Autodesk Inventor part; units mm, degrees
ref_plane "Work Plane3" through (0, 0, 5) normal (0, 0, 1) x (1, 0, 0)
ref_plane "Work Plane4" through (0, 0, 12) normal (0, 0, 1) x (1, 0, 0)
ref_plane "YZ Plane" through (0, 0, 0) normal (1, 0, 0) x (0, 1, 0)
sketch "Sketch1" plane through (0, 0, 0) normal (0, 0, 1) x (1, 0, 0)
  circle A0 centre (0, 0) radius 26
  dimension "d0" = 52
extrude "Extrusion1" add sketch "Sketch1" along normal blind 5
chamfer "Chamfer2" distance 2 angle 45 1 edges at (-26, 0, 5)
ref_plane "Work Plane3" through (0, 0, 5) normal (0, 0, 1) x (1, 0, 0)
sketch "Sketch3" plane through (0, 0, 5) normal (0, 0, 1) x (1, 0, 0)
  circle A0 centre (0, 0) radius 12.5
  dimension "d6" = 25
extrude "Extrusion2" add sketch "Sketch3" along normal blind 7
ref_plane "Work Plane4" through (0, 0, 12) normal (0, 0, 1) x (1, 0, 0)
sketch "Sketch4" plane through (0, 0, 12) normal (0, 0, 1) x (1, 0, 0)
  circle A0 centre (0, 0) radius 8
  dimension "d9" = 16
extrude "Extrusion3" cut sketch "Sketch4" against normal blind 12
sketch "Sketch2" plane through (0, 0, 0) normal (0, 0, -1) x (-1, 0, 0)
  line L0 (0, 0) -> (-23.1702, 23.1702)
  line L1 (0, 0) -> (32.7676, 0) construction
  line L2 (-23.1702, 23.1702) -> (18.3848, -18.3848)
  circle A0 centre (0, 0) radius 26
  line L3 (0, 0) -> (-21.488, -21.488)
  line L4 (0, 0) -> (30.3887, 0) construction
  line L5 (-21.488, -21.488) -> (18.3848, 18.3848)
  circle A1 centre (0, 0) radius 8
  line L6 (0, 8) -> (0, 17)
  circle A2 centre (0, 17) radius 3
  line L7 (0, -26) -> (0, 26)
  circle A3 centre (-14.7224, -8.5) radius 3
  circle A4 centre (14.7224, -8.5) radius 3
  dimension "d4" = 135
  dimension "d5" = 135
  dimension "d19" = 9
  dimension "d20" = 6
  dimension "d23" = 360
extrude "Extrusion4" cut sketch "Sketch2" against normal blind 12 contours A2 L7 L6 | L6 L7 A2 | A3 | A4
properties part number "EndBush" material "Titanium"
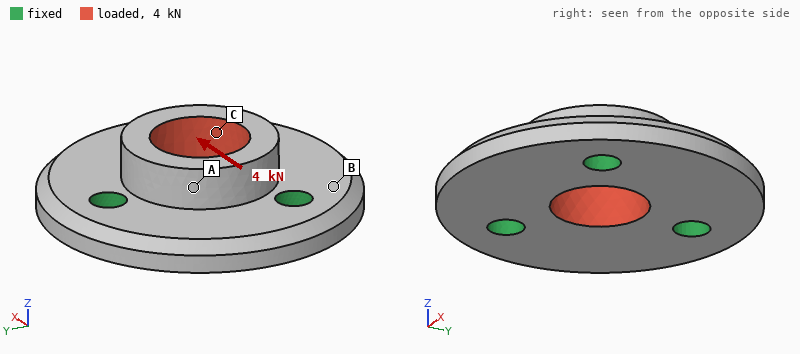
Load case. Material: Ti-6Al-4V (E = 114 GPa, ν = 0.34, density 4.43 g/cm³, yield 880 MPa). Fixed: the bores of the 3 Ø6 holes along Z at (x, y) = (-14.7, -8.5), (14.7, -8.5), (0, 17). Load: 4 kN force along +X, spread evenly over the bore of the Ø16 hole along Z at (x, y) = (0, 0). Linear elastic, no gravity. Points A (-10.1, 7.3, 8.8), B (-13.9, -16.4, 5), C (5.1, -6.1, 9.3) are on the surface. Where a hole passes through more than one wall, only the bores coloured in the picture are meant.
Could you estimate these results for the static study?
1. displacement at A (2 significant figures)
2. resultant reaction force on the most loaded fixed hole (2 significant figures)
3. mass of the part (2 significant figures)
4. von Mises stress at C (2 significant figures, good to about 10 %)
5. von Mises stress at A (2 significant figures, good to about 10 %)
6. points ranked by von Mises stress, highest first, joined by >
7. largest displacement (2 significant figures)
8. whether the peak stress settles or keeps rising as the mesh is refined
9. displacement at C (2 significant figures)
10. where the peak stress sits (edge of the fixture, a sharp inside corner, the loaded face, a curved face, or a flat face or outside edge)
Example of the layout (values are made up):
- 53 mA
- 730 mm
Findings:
- 4.3 µm
- 1.4 kN
- 48 g
- 22 MPa
- 11 MPa
- C > A > B
- 5.5 µm
- keeps rising
- 2.7 µm
- edge of the fixture
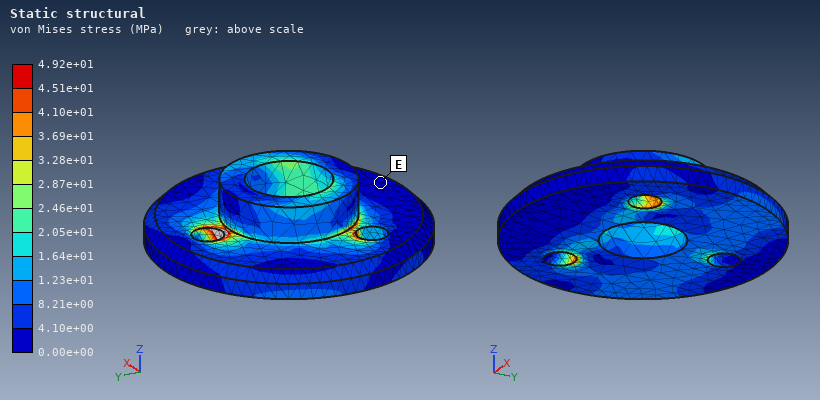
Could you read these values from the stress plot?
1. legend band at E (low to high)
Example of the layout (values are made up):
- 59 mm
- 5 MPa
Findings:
- 0.00e+00 to 4.10e+00 MPa
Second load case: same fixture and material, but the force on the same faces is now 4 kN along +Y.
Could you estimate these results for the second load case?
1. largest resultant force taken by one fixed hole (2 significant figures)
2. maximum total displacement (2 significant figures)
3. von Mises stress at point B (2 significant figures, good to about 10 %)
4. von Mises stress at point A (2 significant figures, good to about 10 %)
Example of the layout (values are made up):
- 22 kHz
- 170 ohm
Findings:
- 1.4 kN
- 6.1 µm
- 10 MPa
- 10 MPa
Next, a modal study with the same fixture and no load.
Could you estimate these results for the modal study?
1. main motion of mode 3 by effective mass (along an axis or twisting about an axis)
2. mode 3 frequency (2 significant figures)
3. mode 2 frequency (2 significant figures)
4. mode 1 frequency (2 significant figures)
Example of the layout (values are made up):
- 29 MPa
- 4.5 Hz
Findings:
- along Z
- 18 kHz
- 16 kHz
- 16 kHz
